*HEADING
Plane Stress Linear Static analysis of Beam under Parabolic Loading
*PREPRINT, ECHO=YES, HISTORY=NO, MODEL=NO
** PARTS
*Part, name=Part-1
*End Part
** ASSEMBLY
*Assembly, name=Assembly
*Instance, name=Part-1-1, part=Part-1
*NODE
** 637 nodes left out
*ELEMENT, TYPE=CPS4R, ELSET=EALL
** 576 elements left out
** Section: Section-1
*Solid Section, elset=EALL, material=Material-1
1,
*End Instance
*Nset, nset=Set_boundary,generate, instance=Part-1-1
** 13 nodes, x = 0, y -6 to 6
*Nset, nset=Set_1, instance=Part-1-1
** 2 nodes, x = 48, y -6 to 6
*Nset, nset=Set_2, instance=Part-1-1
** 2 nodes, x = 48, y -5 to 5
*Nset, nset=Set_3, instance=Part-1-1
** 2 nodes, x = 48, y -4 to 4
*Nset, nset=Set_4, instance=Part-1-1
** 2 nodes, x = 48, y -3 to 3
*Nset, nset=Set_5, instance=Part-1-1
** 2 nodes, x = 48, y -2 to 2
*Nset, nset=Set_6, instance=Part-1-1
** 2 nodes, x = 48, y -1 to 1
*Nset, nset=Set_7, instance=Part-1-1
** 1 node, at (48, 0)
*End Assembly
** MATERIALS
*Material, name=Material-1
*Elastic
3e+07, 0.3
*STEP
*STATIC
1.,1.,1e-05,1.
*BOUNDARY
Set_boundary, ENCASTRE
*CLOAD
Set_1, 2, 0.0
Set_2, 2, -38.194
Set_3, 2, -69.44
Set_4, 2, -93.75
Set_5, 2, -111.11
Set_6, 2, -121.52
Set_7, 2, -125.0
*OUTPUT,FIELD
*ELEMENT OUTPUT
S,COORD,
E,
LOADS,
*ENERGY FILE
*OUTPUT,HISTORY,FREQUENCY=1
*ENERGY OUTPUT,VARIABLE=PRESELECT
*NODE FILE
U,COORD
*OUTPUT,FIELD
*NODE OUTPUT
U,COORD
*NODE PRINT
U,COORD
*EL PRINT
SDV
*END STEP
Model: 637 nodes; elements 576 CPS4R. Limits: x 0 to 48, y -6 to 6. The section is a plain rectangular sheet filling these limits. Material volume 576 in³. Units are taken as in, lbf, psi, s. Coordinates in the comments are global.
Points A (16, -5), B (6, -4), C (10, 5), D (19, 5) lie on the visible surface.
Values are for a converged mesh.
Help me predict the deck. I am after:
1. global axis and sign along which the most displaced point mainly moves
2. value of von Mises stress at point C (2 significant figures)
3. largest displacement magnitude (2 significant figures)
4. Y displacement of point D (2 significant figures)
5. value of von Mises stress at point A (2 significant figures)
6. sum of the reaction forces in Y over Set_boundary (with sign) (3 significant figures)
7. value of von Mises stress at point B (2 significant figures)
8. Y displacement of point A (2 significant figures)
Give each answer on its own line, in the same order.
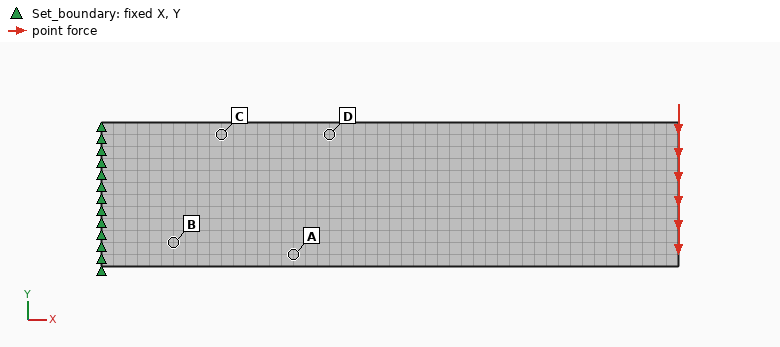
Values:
-Y
1300 psi
0.0090 in
-0.0019 in
1100 psi
993 lbf
1200 psi
-0.0014 in
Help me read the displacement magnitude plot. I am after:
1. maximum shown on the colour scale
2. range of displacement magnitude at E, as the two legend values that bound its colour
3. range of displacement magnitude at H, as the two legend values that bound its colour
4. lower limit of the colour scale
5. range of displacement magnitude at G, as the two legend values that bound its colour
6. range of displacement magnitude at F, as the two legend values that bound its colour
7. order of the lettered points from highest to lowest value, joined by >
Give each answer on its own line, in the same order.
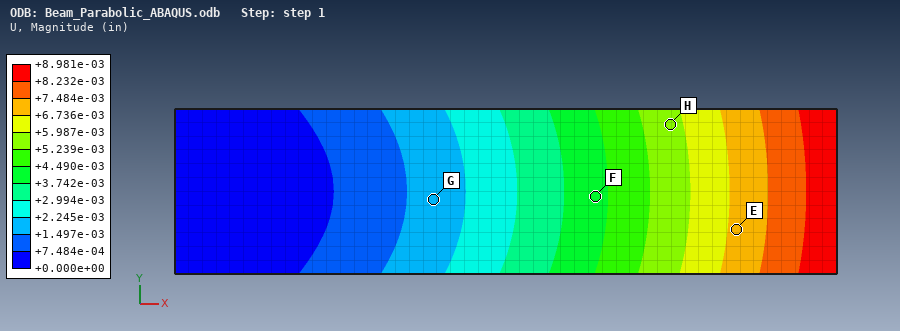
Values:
+8.981e-03 in
+6.736e-03 to +7.484e-03 in
+5.239e-03 to +5.987e-03 in
+0.000e+00 in
+1.497e-03 to +2.245e-03 in
+3.742e-03 to +4.490e-03 in
E > H > F > G
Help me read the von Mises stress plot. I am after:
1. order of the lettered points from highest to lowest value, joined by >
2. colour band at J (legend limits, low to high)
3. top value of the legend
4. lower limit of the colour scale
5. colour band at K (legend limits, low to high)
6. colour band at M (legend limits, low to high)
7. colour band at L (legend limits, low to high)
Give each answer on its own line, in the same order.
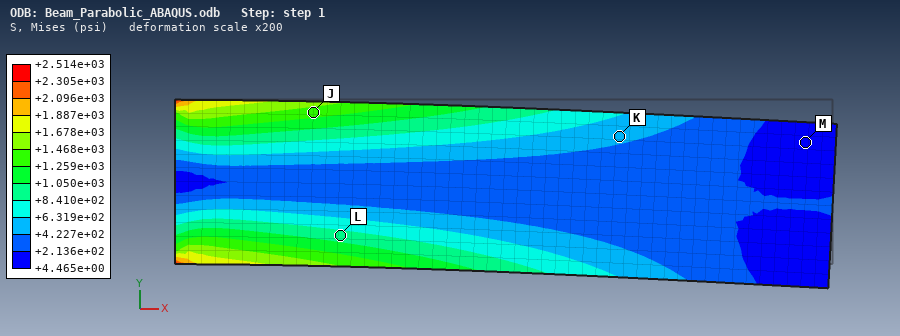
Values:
J > L > K > M
+1.259e+03 to +1.468e+03 psi
+2.514e+03 psi
+4.465e+00 psi
+4.227e+02 to +6.319e+02 psi
+4.465e+00 to +2.136e+02 psi
+8.410e+02 to +1.050e+03 psi
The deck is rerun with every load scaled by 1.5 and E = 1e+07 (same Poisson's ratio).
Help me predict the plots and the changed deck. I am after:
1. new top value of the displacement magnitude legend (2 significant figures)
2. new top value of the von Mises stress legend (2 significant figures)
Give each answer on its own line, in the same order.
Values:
0.040 in
3800 psi
